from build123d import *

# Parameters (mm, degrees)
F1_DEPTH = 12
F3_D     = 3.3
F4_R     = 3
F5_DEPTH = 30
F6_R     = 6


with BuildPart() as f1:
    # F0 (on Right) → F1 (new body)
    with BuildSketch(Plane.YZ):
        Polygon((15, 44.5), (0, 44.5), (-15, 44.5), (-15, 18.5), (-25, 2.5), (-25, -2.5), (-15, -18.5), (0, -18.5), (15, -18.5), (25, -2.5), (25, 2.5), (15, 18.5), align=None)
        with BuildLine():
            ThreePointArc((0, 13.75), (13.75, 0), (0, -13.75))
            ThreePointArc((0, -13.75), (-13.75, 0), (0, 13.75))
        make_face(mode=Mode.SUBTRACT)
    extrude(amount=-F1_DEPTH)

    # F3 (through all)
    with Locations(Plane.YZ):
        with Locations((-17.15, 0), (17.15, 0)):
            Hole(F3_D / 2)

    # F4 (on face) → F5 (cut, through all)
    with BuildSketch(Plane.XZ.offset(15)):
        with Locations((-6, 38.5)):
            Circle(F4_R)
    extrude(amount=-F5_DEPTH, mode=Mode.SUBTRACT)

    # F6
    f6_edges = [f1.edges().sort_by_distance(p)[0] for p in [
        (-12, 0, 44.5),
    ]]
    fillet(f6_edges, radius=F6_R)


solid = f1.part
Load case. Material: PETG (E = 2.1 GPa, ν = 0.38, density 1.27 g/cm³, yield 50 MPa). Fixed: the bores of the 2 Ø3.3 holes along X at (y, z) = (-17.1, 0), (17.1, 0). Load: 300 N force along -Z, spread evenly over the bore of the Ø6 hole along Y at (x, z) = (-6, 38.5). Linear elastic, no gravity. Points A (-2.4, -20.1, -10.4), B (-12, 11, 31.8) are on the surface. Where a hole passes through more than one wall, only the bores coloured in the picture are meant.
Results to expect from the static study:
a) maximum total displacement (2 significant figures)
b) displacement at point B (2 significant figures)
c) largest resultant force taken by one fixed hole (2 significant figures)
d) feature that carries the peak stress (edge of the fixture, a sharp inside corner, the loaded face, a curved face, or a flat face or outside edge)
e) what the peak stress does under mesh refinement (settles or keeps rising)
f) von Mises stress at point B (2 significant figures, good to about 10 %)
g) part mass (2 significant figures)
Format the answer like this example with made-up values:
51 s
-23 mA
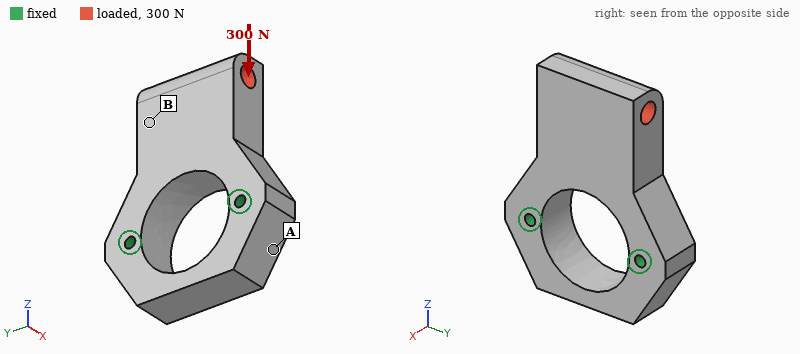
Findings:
30 µm
22 µm
160 N
edge of the fixture
keeps rising
1.1 MPa
25 g
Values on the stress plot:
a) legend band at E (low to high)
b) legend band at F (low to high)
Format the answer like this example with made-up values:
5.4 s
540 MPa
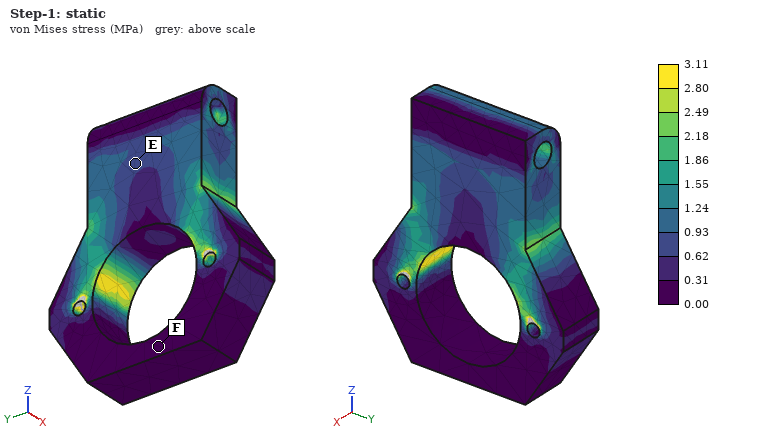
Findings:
0.62 to 0.93 MPa
0.00 to 0.31 MPa
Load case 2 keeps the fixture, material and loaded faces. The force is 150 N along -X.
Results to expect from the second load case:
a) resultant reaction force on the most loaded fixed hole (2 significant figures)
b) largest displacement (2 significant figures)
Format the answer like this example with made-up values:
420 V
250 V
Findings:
75 N
0.74 mm
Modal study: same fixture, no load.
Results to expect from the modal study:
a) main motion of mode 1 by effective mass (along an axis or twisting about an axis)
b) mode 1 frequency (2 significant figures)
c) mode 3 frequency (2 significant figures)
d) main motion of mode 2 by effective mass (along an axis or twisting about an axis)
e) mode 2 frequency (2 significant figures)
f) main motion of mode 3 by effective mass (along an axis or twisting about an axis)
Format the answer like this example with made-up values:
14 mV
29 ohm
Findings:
along X
980 Hz
3300 Hz
along Y
2900 Hz
twisting about Z
